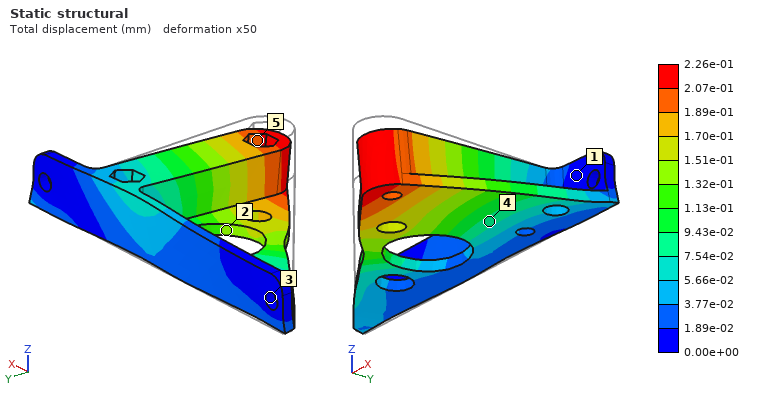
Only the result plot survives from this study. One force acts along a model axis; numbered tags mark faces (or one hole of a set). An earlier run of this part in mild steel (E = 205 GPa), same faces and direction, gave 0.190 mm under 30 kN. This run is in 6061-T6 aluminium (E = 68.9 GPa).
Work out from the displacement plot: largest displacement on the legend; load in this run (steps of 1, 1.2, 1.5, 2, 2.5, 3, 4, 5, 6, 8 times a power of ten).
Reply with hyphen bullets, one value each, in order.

- 2.26e-01 mm
- 12 kN
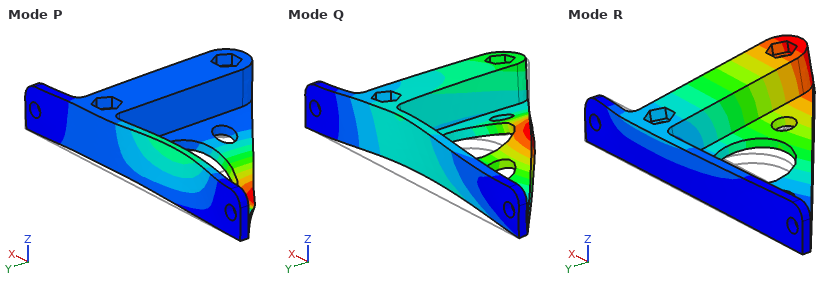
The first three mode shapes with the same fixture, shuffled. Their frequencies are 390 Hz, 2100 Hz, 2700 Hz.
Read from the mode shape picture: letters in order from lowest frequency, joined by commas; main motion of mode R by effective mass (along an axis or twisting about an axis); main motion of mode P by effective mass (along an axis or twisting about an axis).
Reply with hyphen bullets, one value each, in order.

- R, Q, P
- along Z
- along Y
